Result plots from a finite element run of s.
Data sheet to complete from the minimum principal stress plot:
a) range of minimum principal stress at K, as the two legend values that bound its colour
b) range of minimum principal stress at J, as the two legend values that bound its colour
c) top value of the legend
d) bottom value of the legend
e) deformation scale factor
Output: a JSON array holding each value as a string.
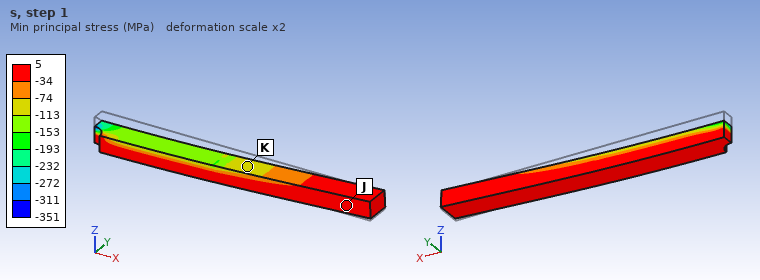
["-113 to -74 MPa", "-34 to 5 MPa", "5 MPa", "-351 MPa", "2"]
